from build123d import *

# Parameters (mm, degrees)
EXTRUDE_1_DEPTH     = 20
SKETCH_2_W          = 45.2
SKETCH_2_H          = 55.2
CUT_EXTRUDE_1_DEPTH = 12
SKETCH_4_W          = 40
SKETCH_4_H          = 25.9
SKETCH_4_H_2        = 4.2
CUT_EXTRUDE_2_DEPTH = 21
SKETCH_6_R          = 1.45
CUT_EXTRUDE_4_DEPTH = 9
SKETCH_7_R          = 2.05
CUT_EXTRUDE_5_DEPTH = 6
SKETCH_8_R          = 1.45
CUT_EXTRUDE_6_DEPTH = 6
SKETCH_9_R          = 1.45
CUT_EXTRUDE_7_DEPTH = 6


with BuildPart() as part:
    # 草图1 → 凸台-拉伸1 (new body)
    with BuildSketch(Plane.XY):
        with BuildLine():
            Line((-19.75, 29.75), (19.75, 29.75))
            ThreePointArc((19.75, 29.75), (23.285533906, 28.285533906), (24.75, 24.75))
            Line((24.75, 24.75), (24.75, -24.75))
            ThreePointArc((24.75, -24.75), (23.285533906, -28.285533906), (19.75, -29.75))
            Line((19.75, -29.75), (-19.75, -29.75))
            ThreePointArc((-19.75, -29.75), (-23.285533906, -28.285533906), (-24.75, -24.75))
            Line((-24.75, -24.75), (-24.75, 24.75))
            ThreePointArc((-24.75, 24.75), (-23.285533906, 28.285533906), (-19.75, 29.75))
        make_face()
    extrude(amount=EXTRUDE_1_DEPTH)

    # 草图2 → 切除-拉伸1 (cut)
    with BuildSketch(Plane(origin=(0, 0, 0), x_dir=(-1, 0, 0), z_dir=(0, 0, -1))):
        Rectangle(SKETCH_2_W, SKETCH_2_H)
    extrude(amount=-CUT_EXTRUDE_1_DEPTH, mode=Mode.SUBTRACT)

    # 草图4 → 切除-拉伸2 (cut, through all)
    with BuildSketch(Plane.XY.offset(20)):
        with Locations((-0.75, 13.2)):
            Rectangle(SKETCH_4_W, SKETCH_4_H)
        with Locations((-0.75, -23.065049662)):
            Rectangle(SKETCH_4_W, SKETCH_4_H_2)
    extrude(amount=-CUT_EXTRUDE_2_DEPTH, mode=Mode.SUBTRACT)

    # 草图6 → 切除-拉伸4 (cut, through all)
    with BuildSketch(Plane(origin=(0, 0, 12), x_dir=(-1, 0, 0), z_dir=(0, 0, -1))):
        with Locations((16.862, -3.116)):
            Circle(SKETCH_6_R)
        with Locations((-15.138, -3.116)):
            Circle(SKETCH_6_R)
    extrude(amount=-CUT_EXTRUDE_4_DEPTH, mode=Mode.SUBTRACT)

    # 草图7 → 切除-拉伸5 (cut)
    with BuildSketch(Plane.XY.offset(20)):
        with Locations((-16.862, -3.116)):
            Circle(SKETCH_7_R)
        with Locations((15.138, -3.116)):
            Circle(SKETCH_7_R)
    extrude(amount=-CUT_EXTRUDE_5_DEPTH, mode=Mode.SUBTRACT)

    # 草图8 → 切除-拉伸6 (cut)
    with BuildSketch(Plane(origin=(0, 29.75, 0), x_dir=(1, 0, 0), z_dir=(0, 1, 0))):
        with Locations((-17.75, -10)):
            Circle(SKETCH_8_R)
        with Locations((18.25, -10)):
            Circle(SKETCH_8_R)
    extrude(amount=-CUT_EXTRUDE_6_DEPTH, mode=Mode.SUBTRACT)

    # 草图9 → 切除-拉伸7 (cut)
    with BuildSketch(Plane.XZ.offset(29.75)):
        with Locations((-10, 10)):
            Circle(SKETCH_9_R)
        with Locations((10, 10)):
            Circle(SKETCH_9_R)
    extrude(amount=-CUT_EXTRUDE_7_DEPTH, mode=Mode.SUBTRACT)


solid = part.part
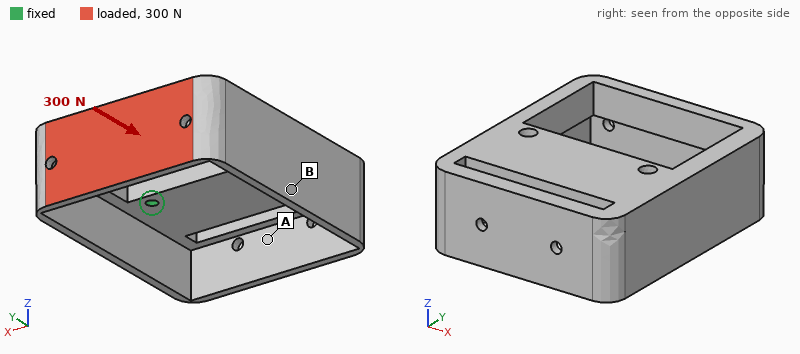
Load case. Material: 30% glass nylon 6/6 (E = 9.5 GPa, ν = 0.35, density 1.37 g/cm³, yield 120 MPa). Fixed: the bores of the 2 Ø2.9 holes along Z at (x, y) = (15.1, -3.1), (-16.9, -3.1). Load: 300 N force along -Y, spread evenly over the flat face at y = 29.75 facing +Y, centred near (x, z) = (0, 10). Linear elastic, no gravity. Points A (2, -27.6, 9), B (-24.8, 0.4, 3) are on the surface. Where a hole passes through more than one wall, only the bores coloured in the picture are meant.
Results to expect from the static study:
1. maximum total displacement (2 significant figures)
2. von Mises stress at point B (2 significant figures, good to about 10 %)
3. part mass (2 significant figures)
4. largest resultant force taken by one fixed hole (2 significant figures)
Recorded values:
0.76 mm
8.3 MPa
26 g
180 N
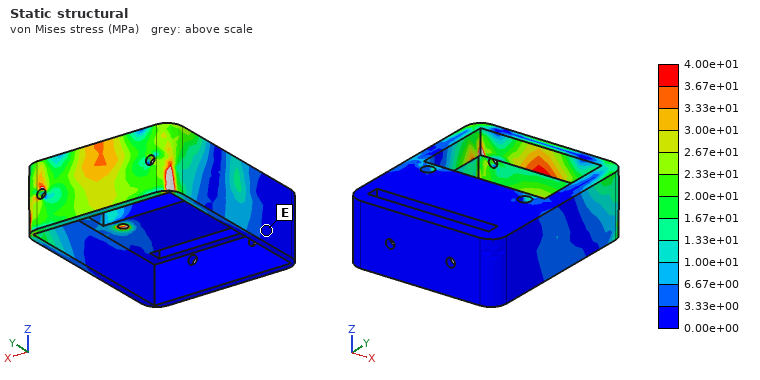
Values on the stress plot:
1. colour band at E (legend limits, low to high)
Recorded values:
0.00e+00 to 3.33e+00 MPa
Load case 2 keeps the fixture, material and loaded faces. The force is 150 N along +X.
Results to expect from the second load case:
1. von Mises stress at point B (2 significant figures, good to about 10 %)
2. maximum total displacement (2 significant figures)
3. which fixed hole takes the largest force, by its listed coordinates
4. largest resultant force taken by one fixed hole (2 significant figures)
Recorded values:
9.9 MPa
0.54 mm
(15.1, -3.1)
180 N
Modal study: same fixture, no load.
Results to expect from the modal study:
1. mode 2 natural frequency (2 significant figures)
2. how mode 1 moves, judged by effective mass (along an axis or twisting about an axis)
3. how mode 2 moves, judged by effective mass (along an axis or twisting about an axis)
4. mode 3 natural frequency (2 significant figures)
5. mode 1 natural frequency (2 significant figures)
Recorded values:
1300 Hz
twisting about X
along X
2300 Hz
770 Hz
